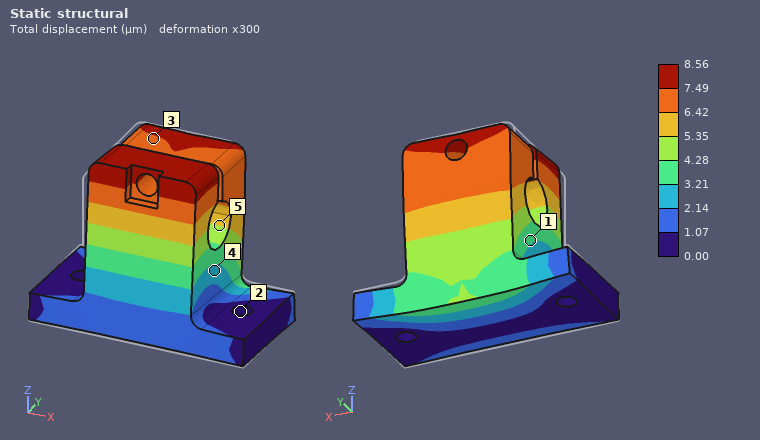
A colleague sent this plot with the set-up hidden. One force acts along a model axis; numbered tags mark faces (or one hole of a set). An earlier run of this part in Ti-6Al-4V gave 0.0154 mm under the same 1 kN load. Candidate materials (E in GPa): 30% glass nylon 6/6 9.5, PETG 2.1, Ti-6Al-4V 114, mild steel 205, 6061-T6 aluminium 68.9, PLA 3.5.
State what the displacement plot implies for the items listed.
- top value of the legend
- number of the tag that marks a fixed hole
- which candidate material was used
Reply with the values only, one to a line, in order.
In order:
8.56 µm
2
mild steel
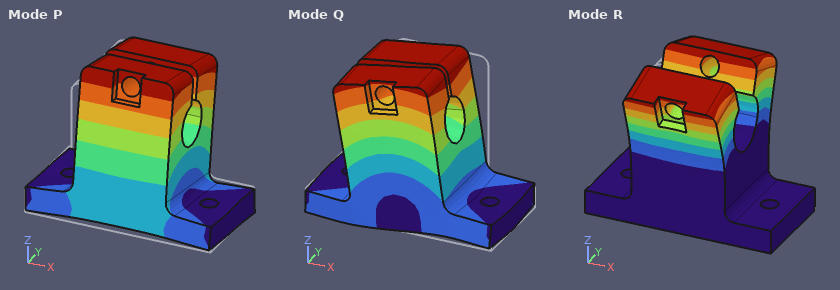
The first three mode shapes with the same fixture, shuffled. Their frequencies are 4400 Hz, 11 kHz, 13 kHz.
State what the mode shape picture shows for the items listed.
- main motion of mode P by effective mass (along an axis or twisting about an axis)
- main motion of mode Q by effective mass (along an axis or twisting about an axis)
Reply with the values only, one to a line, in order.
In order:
along Y
along X
